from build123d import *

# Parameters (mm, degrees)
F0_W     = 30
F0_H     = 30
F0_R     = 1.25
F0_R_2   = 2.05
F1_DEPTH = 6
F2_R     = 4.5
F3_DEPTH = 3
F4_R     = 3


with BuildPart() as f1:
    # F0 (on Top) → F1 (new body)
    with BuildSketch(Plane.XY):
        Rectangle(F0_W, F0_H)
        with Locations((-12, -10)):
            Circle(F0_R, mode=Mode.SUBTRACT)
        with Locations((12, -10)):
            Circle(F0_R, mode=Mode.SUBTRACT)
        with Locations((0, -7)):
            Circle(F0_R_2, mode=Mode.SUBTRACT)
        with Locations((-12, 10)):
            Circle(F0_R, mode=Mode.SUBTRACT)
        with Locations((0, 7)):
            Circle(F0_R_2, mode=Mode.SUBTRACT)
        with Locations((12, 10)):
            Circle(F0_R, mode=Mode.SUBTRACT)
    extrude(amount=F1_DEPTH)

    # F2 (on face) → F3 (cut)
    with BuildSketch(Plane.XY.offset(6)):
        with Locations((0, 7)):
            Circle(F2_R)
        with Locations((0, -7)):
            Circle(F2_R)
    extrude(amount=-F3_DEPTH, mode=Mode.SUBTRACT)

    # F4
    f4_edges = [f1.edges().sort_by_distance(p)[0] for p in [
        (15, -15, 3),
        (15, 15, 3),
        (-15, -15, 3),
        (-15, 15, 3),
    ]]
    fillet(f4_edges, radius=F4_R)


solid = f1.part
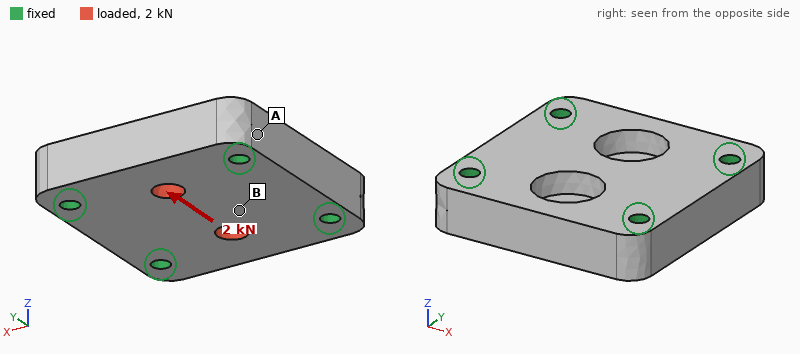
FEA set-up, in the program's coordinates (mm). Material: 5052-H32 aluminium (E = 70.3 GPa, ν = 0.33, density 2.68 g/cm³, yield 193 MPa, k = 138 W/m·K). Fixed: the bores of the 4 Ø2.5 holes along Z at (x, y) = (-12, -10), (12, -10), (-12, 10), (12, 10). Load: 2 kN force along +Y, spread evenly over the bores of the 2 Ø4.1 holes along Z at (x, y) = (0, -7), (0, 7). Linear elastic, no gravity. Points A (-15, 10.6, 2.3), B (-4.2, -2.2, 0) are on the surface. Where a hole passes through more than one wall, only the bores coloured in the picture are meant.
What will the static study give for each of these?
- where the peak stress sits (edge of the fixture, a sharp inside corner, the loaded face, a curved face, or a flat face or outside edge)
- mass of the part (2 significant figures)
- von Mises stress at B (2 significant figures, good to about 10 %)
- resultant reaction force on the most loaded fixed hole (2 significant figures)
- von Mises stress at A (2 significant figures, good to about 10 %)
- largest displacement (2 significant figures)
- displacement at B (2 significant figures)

the loaded face
13 g
19 MPa
540 N
8.3 MPa
4.8 µm
2.7 µm
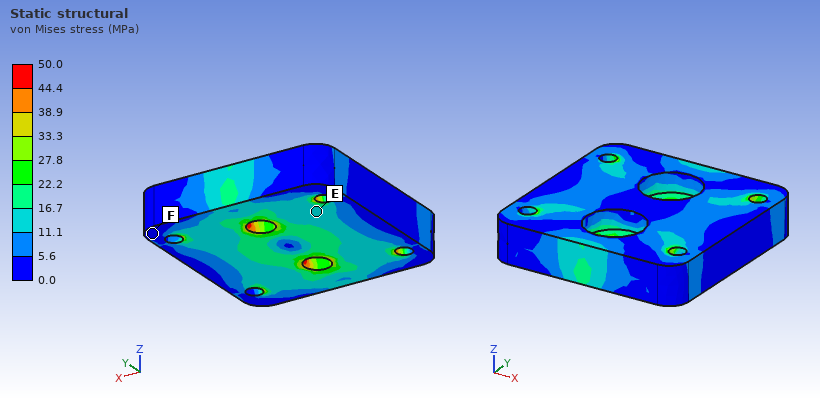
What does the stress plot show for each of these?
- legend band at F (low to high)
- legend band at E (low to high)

0.0 to 5.6 MPa
11.1 to 16.7 MPa
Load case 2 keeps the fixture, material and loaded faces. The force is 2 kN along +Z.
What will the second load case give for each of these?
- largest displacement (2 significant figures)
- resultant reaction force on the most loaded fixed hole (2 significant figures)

17 µm
530 N
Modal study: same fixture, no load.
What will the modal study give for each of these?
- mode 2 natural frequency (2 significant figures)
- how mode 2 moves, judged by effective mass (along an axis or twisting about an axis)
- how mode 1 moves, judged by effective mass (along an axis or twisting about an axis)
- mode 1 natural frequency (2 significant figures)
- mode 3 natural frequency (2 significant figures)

44 kHz
twisting about X
along Z
34 kHz
48 kHz
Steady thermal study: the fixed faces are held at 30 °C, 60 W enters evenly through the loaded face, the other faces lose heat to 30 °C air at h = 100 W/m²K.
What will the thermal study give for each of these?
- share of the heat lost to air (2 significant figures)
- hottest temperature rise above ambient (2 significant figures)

3.3 %
25 K
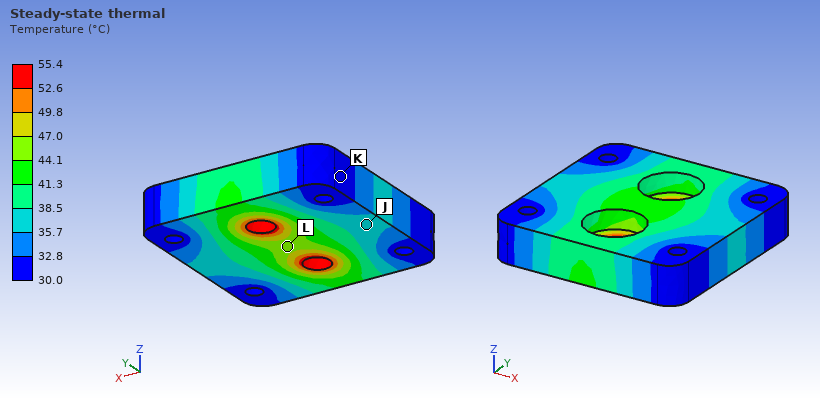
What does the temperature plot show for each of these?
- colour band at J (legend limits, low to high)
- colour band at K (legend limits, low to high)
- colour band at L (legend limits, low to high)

35.7 to 38.5 °C
30.0 to 32.8 °C
44.1 to 47.0 °C
